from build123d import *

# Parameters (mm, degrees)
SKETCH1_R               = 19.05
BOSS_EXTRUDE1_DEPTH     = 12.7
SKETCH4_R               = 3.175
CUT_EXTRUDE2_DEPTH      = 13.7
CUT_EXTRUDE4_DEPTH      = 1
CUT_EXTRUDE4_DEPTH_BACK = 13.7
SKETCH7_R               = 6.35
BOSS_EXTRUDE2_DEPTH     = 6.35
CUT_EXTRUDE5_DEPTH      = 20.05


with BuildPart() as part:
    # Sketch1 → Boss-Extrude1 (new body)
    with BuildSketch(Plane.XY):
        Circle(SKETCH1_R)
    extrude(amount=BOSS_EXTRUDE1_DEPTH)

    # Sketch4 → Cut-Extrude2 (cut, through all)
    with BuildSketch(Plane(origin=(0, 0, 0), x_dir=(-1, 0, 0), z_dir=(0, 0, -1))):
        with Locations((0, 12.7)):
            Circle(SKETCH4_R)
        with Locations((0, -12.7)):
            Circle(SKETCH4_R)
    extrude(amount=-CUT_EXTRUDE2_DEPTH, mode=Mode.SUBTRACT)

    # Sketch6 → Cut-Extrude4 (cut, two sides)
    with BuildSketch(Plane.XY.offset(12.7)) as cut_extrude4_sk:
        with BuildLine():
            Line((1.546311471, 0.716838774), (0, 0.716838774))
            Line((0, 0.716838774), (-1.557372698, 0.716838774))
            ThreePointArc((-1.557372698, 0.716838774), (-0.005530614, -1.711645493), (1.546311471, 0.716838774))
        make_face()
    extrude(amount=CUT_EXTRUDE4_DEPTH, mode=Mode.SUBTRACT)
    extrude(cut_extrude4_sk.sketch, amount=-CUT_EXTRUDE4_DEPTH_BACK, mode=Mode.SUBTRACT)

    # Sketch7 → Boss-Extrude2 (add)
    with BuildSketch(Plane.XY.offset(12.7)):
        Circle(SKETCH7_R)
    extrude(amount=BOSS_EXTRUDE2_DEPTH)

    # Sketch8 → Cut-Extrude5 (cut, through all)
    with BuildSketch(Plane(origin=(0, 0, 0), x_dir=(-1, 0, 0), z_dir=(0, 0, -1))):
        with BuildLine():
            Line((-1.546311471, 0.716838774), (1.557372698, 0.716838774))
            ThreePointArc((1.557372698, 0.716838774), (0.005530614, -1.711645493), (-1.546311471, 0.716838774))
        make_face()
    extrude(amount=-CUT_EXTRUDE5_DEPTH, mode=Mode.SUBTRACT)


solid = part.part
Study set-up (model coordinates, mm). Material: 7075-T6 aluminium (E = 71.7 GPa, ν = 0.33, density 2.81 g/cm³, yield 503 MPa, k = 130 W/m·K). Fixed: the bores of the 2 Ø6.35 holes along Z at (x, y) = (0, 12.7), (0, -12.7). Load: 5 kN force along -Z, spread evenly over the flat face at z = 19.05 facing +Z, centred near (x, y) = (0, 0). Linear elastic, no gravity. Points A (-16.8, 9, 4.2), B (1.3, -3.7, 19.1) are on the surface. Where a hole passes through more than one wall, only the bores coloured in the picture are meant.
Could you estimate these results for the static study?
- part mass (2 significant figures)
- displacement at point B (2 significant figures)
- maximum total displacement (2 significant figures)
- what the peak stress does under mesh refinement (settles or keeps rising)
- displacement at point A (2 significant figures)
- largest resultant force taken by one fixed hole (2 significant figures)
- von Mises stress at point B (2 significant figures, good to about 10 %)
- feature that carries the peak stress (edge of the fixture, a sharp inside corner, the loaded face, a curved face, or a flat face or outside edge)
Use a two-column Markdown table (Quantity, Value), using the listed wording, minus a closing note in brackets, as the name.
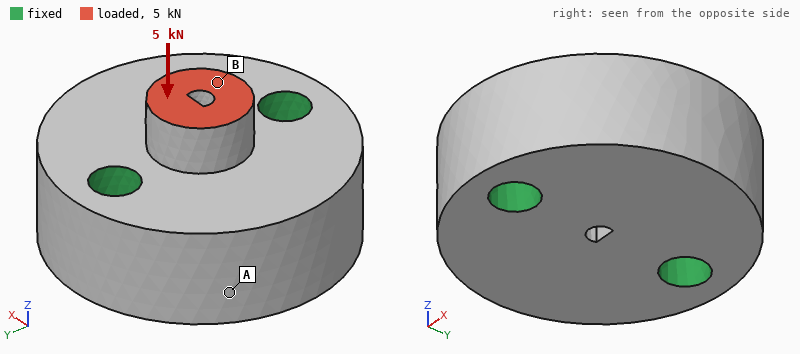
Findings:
| Quantity | Value |
|---|---|
| part mass | 40 g |
| displacement at point B | 8.6 µm |
| maximum total displacement | 8.9 µm |
| what the peak stress does under mesh refinement | keeps rising |
| displacement at point A | 2.7 µm |
| largest resultant force taken by one fixed hole | 2.5 kN |
| von Mises stress at point B | 43 MPa |
| feature that carries the peak stress | edge of the fixture |
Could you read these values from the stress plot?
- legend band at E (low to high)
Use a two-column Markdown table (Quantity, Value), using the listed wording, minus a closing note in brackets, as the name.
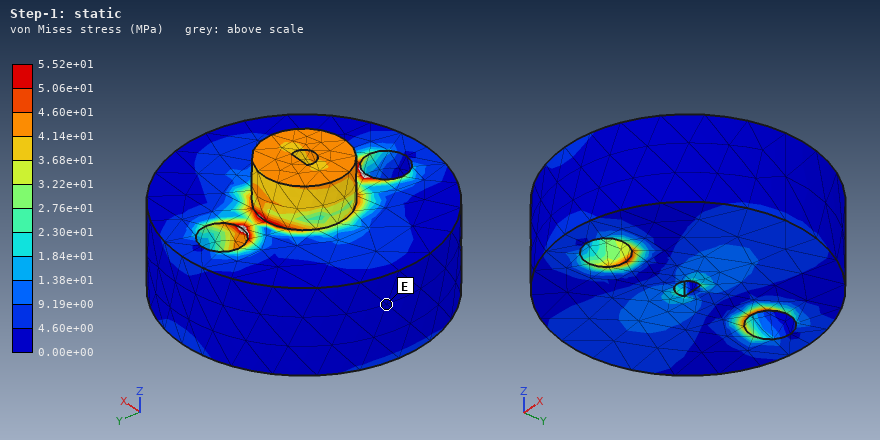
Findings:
| Quantity | Value |
|---|---|
| legend band at E | 0.00e+00 to 4.60e+00 MPa |
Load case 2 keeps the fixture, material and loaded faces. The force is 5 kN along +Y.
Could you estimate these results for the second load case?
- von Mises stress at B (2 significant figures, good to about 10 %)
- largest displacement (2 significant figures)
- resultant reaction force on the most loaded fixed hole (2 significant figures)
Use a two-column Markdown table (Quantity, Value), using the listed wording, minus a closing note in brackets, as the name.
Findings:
| Quantity | Value |
|---|---|
| von Mises stress at B | 98 MPa |
| largest displacement | 35 µm |
| resultant reaction force on the most loaded fixed hole | 3.6 kN |
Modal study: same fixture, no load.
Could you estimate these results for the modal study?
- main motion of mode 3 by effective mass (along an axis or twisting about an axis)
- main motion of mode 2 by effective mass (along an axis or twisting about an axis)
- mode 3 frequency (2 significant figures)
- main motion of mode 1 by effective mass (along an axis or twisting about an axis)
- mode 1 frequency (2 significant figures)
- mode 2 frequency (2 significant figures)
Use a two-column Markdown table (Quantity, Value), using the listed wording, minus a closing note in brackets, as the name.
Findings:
| Quantity | Value |
|---|---|
| main motion of mode 3 by effective mass | along Y |
| main motion of mode 2 by effective mass | along Z |
| mode 3 frequency | 46 kHz |
| main motion of mode 1 by effective mass | twisting about Y |
| mode 1 frequency | 24 kHz |
| mode 2 frequency | 29 kHz |
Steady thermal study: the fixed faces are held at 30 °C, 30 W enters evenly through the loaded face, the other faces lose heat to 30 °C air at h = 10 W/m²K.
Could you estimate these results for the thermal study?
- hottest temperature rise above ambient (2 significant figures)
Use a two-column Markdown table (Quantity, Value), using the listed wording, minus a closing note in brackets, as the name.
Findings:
| Quantity | Value |
|---|---|
| hottest temperature rise above ambient | 20 K |
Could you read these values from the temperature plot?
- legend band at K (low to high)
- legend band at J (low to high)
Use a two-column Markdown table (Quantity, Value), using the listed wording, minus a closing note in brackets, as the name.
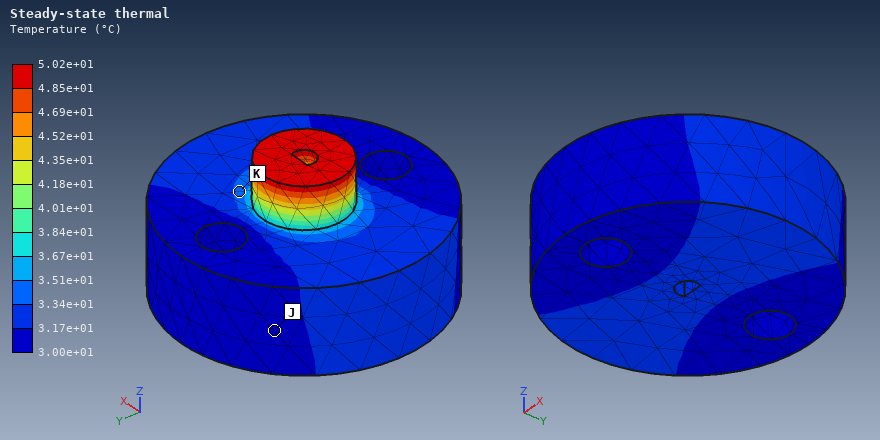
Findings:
| Quantity | Value |
|---|---|
| legend band at K | 3.34e+01 to 3.51e+01 °C |
| legend band at J | 3.00e+01 to 3.17e+01 °C |
